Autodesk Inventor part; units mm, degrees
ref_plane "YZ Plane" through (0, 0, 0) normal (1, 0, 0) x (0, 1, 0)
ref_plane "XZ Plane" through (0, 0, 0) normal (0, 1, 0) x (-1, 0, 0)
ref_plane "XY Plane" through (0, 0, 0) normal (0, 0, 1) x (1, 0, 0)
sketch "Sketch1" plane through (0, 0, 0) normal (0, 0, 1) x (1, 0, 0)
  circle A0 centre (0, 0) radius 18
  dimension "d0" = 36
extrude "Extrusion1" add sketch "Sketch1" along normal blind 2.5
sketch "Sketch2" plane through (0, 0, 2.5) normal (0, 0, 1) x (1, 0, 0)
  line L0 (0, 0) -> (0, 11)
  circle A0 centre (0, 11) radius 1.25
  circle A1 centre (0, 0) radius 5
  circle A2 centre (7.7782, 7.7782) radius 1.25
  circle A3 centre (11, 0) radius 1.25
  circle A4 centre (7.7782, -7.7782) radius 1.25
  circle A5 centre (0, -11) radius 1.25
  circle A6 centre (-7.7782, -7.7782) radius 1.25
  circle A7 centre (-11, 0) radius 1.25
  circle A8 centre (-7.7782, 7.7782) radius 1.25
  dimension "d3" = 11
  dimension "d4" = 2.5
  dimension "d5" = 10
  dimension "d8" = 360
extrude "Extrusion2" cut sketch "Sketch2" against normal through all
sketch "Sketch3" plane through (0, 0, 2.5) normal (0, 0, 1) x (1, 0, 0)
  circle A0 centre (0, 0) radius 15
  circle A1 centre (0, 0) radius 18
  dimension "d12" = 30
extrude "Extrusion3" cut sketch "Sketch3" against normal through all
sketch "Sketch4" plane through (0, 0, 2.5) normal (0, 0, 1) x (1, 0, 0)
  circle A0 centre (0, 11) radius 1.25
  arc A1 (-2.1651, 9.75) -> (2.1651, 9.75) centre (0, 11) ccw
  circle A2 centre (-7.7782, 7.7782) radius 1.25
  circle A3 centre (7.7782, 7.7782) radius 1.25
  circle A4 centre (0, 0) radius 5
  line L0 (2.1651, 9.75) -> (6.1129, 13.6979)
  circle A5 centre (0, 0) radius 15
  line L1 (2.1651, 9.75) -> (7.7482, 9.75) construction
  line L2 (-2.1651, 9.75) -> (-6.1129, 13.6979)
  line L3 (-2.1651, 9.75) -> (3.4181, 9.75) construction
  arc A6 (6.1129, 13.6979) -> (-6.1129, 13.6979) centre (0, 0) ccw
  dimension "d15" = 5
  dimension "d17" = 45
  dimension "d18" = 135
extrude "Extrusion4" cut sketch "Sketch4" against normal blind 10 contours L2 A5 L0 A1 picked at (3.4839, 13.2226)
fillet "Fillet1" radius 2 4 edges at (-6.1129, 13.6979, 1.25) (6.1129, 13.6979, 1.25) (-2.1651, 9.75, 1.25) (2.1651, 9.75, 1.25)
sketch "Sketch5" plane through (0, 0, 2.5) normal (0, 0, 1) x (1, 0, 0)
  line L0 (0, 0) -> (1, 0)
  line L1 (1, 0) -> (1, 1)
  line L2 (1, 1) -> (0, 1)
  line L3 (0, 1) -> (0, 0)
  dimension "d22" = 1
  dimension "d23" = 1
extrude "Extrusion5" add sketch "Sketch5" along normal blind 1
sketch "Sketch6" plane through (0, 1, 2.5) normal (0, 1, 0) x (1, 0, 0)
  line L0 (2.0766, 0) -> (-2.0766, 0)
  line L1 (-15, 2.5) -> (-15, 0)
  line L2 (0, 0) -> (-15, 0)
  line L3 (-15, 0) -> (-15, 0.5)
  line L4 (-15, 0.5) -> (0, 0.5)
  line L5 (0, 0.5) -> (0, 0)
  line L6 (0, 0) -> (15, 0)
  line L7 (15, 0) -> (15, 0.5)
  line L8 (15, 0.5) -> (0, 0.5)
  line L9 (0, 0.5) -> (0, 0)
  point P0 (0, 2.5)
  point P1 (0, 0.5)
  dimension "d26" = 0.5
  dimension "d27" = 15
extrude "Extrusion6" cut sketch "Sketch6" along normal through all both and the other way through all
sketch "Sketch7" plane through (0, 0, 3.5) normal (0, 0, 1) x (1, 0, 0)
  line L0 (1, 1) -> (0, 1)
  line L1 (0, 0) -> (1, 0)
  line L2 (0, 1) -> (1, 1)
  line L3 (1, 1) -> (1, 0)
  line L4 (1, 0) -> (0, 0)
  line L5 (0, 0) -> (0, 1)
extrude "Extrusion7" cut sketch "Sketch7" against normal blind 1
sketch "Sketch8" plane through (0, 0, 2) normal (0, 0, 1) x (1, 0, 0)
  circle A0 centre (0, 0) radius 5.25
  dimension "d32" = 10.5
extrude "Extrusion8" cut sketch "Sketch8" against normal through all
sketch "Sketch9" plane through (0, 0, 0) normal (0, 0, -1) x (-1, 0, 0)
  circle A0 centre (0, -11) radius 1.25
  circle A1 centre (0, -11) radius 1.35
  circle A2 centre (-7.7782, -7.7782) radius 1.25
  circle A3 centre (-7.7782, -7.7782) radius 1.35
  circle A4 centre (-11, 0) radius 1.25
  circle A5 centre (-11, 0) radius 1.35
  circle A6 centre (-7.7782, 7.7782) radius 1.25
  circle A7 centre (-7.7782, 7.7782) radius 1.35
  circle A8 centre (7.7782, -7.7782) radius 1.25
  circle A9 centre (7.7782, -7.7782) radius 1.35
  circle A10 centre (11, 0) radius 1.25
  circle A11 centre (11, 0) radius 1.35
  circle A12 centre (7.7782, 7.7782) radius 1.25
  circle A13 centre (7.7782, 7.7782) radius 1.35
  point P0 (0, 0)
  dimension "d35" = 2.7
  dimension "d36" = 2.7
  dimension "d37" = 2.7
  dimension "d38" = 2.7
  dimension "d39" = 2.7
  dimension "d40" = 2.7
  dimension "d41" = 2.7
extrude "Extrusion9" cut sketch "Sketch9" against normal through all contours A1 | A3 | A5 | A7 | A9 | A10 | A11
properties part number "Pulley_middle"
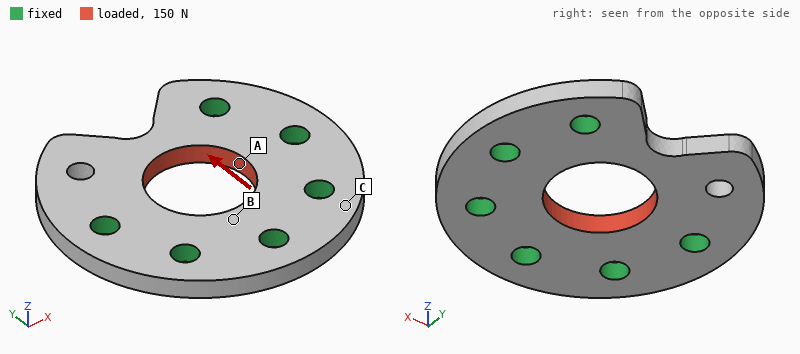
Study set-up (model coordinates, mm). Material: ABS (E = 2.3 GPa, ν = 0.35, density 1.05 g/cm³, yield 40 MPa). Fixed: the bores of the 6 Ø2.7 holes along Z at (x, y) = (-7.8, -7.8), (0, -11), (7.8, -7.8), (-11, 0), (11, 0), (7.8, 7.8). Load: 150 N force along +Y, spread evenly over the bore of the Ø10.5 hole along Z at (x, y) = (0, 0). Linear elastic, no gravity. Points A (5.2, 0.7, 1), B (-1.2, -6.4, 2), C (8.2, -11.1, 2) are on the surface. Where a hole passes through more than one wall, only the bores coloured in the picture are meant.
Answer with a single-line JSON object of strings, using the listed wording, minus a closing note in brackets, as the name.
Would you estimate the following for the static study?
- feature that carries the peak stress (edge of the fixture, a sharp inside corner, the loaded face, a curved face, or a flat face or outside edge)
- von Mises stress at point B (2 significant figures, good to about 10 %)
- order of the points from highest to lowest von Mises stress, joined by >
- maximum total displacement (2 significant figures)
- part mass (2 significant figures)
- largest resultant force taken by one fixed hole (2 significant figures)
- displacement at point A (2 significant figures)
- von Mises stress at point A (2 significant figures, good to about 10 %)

{"feature that carries the peak stress": "a curved face", "von Mises stress at point B": "2.3 MPa", "order of the points from highest to lowest von Mises stress, joined by >": "A > B > C", "maximum total displacement": "29 µm", "part mass": "1.1 g", "largest resultant force taken by one fixed hole": "33 N", "displacement at point A": "7.9 µm", "von Mises stress at point A": "4.2 MPa"}
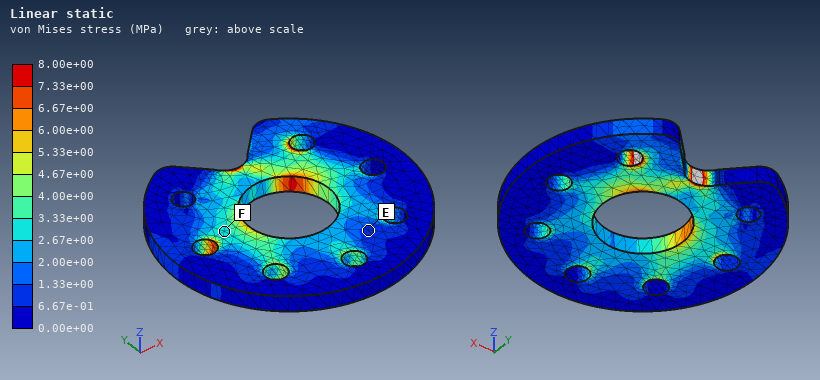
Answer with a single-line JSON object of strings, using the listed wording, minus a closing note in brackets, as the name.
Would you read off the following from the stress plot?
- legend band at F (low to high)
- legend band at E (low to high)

{"legend band at F": "2.67e+00 to 3.33e+00 MPa", "legend band at E": "6.67e-01 to 1.33e+00 MPa"}
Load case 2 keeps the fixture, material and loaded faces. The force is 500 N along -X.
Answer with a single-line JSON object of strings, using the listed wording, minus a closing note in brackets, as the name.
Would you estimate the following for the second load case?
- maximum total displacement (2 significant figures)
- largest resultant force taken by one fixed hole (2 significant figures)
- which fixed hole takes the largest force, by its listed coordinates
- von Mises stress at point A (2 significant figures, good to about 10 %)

{"maximum total displacement": "48 µm", "largest resultant force taken by one fixed hole": "130 N", "which fixed hole takes the largest force, by its listed coordinates": "(-11, 0)", "von Mises stress at point A": "6.9 MPa"}
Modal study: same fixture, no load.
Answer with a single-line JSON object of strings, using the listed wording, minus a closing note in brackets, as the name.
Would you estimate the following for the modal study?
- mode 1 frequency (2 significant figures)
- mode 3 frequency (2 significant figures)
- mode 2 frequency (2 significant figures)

{"mode 1 frequency": "4400 Hz", "mode 3 frequency": "15 kHz", "mode 2 frequency": "11 kHz"}
